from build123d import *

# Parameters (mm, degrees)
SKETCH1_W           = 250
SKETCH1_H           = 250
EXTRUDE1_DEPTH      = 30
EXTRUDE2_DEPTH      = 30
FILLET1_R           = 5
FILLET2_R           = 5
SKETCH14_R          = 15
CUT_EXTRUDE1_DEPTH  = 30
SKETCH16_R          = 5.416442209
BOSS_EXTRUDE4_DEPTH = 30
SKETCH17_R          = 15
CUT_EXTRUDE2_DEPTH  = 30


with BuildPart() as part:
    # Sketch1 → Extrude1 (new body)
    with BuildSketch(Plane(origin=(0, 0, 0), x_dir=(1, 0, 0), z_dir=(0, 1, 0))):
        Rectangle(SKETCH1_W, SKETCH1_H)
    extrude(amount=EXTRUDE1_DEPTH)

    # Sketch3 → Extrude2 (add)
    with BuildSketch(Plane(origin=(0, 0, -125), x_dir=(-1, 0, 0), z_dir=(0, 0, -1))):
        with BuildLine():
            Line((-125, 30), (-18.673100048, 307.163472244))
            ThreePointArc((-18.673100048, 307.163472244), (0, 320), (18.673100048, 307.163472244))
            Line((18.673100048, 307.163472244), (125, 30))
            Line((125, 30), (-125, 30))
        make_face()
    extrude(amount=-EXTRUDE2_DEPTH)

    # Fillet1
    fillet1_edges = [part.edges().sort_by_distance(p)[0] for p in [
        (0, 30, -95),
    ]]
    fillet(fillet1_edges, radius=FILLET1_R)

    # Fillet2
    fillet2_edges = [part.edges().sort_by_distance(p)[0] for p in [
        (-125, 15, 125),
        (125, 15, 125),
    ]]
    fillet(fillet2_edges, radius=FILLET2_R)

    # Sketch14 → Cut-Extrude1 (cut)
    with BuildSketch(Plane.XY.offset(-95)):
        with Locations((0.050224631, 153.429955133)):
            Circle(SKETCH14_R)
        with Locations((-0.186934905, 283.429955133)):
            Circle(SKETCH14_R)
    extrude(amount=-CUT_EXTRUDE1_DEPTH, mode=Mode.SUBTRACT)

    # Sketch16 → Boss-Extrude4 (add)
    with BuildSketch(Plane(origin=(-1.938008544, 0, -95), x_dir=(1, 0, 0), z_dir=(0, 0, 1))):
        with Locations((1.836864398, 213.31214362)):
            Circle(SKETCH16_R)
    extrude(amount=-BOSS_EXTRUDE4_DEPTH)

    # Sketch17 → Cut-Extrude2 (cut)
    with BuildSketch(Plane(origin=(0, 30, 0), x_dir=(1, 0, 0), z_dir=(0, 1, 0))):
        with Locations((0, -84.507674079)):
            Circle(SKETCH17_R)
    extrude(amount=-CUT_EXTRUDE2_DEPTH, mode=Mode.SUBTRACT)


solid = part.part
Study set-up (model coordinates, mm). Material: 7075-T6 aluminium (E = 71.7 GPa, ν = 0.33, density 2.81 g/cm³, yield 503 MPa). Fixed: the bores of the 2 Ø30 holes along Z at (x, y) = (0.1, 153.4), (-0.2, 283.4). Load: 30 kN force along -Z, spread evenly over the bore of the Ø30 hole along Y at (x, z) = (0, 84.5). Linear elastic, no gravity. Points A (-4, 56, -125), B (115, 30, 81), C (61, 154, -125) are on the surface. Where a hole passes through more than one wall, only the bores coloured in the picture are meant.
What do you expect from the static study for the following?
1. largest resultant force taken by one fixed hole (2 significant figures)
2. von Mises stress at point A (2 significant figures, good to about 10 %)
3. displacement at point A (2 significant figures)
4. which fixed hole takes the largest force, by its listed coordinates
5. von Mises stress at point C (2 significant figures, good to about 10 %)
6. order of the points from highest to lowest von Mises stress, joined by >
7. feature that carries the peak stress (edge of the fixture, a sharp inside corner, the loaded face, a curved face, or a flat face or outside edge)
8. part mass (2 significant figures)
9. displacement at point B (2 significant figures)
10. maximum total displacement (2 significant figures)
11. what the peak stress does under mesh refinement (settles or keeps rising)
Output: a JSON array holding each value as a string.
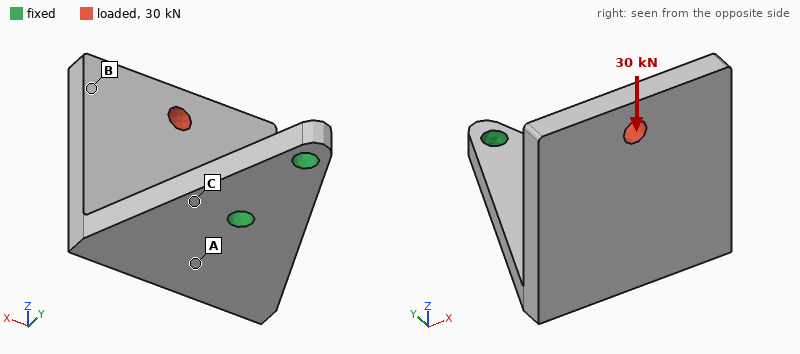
["37 kN", "35 MPa", "0.59 mm", "(0.1, 153.4)", "82 MPa", "C > A > B", "edge of the fixture", "8.5 kg", "2.0 mm", "2.6 mm", "keeps rising"]
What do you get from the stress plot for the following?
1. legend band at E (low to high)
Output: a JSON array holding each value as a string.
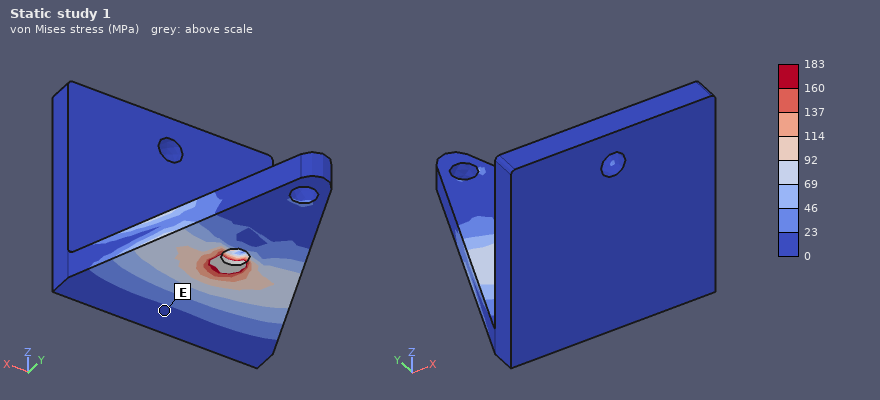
["0 to 23 MPa"]
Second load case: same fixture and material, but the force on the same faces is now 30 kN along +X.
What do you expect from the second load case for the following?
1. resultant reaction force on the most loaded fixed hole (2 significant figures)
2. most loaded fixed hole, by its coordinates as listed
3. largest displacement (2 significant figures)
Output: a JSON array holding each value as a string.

["52 kN", "(0.1, 153.4)", "4.3 mm"]
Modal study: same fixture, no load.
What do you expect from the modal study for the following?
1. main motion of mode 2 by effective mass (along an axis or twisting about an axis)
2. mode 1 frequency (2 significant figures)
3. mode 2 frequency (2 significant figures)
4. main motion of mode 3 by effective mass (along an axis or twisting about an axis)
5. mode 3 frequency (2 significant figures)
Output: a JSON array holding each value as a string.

["along X", "210 Hz", "280 Hz", "along Z", "640 Hz"]
